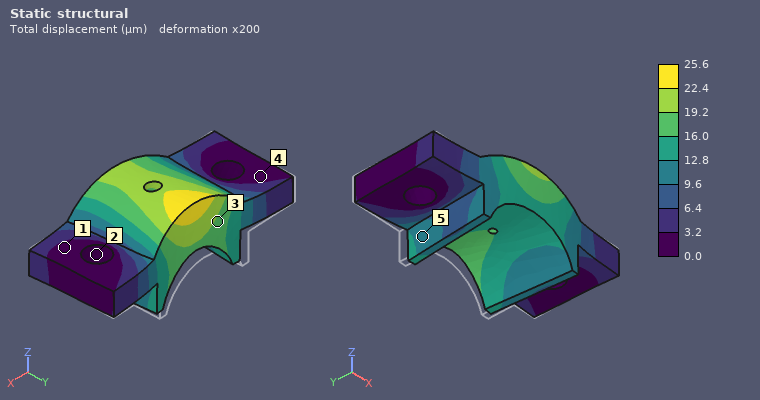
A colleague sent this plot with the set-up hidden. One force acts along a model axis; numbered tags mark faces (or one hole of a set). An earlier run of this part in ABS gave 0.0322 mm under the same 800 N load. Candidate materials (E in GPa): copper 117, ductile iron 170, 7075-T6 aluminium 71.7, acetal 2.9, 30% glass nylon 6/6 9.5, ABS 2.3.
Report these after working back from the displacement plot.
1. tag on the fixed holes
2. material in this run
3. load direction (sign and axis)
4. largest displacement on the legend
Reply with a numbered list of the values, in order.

1. 2
2. acetal
3. -Y
4. 25.6 µm
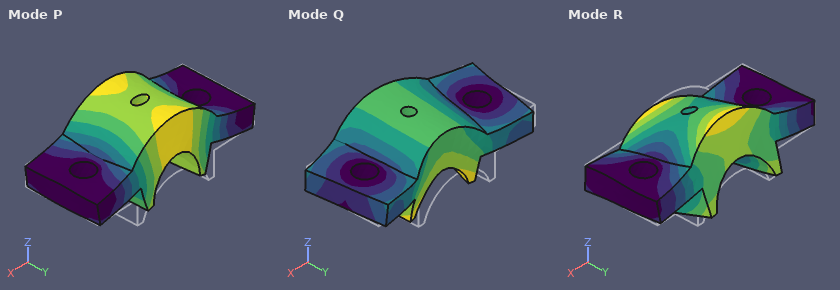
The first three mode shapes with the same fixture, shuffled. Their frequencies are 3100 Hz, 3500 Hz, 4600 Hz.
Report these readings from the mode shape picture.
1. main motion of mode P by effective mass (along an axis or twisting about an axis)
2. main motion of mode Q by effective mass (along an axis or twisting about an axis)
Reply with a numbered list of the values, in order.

1. along Z
2. along Y
